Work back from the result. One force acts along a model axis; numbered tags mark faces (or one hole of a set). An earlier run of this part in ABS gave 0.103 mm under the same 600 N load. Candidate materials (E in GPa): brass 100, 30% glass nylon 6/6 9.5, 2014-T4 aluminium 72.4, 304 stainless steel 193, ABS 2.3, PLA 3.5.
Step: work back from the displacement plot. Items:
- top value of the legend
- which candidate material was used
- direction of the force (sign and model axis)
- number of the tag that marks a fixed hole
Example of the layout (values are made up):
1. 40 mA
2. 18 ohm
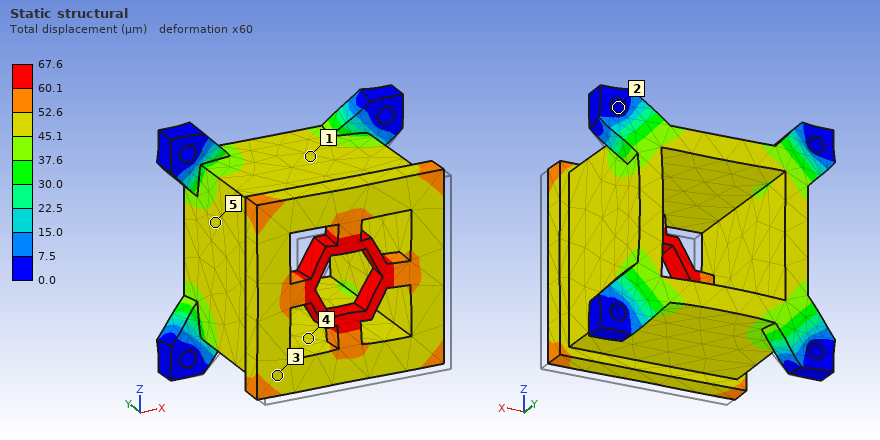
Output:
1. 67.6 µm
2. PLA
3. +Y
4. 2
